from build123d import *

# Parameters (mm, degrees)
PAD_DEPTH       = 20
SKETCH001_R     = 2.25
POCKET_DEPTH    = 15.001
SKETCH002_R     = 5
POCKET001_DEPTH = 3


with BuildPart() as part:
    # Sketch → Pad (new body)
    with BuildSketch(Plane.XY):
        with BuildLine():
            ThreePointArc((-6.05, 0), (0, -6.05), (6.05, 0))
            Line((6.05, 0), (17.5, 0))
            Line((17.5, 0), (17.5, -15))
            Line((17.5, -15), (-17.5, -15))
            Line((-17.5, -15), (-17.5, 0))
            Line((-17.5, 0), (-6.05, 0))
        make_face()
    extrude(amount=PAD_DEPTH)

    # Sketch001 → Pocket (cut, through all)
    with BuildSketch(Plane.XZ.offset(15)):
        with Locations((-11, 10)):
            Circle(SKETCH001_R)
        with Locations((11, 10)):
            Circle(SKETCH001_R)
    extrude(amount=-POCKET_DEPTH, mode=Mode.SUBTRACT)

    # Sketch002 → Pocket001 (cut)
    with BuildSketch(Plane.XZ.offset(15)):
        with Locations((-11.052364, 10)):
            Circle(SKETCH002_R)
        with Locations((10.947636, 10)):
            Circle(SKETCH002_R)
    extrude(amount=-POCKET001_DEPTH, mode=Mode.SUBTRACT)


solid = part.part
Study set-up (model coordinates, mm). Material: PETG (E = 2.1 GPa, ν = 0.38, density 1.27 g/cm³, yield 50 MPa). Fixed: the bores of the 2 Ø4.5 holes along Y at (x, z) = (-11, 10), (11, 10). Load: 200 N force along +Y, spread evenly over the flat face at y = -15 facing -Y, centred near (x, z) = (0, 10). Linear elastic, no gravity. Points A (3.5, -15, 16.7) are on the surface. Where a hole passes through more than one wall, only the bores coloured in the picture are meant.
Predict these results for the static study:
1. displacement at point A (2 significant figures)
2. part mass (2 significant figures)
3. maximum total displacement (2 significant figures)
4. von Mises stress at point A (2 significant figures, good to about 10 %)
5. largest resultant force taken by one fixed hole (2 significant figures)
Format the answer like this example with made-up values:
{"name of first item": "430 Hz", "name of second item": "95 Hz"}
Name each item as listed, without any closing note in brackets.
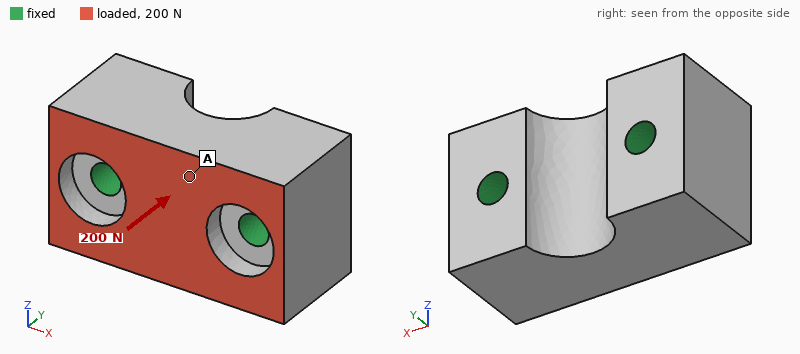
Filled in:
{"displacement at point A": "5.3 µm", "part mass": "11 g", "maximum total displacement": "6.3 µm", "von Mises stress at point A": "0.41 MPa", "largest resultant force taken by one fixed hole": "100 N"}
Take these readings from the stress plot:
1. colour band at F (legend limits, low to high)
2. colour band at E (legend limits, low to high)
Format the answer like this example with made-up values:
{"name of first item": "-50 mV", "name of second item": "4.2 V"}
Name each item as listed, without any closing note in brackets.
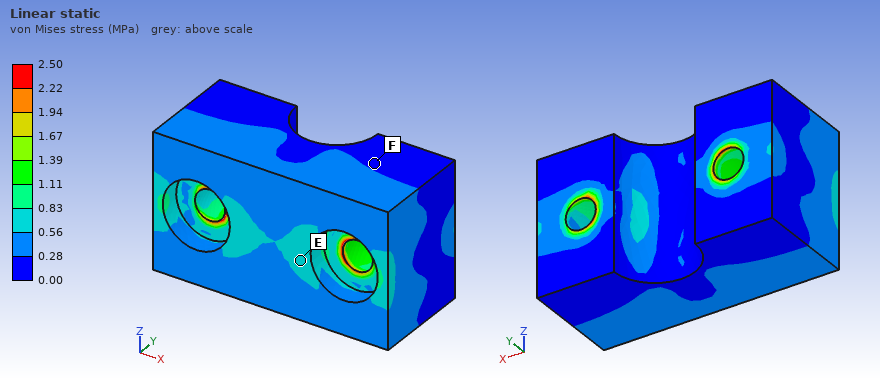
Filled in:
{"colour band at F": "0.00 to 0.28 MPa", "colour band at E": "0.56 to 0.83 MPa"}
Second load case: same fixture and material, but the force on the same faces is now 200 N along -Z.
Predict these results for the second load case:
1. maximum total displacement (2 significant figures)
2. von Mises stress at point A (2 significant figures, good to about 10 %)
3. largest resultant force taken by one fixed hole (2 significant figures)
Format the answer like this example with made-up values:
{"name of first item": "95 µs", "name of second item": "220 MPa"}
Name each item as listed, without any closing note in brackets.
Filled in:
{"maximum total displacement": "19 µm", "von Mises stress at point A": "0.83 MPa", "largest resultant force taken by one fixed hole": "100 N"}
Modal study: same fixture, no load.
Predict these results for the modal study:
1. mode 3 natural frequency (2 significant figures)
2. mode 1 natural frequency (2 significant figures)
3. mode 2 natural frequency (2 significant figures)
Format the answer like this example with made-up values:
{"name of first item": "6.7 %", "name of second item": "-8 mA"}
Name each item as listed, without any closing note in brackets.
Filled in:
{"mode 3 natural frequency": "13 kHz", "mode 1 natural frequency": "9900 Hz", "mode 2 natural frequency": "12 kHz"}
